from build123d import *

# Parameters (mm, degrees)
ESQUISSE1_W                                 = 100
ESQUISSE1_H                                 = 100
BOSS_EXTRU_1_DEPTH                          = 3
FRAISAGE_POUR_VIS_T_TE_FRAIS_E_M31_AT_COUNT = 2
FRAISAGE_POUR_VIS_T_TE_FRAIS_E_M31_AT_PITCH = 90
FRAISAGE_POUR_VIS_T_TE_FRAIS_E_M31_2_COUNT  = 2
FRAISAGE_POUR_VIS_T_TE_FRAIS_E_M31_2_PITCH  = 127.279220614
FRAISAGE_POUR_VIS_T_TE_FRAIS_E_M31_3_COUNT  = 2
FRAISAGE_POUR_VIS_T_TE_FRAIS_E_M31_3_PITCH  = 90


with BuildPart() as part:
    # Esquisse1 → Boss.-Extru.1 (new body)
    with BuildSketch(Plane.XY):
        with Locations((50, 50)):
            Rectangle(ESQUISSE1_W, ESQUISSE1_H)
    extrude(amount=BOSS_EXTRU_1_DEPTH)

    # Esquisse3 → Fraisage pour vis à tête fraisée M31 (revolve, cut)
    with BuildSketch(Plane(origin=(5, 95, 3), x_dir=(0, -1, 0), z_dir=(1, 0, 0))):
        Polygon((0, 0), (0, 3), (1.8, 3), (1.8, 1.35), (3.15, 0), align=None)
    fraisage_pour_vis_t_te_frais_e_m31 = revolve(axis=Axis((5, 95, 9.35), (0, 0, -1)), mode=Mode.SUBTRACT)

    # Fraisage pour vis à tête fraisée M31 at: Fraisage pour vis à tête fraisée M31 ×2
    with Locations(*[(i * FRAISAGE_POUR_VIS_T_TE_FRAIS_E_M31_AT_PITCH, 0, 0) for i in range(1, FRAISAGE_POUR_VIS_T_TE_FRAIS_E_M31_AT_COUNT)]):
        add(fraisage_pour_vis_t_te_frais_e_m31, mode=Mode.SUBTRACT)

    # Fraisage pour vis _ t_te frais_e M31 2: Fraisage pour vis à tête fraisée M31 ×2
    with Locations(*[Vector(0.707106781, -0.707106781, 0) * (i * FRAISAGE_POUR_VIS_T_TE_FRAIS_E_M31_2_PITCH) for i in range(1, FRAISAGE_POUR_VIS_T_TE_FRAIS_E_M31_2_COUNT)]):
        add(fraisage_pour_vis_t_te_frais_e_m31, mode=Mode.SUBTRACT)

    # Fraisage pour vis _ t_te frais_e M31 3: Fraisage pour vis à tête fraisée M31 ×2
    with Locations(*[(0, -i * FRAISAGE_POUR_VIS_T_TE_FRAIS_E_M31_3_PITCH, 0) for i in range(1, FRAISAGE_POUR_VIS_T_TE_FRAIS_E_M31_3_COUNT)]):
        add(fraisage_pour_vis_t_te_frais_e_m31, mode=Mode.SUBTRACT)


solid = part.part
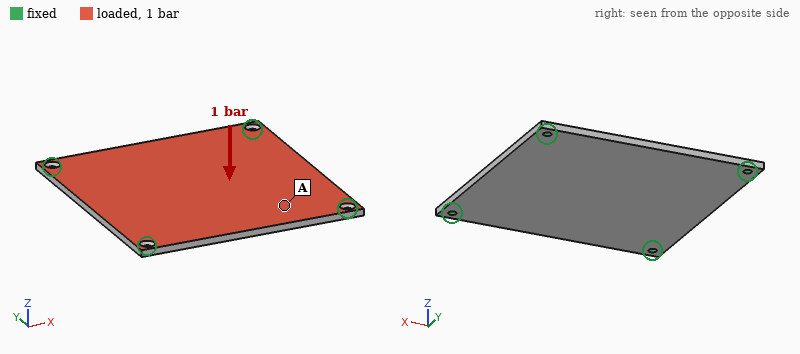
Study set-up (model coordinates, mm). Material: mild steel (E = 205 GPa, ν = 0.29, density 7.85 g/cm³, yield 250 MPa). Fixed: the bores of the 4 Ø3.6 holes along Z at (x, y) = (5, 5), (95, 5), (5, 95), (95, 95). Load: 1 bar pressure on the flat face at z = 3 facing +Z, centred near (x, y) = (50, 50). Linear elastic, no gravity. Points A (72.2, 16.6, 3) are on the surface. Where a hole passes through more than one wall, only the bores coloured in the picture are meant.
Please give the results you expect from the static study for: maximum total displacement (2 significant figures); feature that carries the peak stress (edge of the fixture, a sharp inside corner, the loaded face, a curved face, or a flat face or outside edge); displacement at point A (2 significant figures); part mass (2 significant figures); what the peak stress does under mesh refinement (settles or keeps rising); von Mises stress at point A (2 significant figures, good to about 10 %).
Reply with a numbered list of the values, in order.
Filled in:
1. 0.13 mm
2. edge of the fixture
3. 0.071 mm
4. 230 g
5. keeps rising
6. 23 MPa
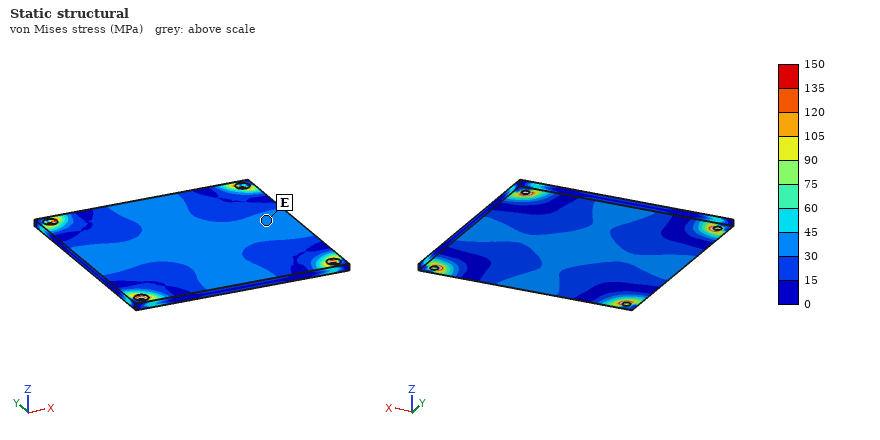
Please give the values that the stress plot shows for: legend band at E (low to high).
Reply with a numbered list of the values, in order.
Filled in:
1. 30 to 45 MPa
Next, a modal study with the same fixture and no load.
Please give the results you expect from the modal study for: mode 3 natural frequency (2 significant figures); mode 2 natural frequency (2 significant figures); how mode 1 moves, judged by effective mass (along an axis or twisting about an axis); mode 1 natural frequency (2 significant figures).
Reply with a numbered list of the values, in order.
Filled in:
1. 2000 Hz
2. 2000 Hz
3. along Z
4. 1100 Hz
